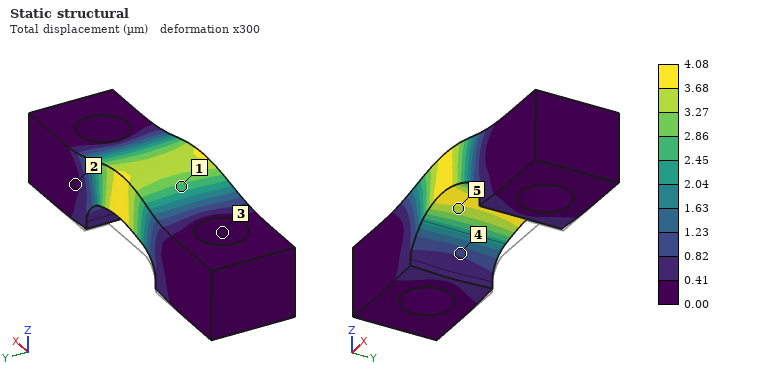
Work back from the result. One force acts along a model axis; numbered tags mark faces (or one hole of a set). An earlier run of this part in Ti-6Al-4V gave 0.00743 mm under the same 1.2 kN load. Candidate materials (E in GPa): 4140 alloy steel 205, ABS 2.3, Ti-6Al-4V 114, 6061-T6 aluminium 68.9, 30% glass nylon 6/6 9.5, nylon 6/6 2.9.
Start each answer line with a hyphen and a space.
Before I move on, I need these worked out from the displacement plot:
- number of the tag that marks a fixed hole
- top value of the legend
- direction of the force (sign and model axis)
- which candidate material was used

- 3
- 4.08 µm
- +Z
- 4140 alloy steel
